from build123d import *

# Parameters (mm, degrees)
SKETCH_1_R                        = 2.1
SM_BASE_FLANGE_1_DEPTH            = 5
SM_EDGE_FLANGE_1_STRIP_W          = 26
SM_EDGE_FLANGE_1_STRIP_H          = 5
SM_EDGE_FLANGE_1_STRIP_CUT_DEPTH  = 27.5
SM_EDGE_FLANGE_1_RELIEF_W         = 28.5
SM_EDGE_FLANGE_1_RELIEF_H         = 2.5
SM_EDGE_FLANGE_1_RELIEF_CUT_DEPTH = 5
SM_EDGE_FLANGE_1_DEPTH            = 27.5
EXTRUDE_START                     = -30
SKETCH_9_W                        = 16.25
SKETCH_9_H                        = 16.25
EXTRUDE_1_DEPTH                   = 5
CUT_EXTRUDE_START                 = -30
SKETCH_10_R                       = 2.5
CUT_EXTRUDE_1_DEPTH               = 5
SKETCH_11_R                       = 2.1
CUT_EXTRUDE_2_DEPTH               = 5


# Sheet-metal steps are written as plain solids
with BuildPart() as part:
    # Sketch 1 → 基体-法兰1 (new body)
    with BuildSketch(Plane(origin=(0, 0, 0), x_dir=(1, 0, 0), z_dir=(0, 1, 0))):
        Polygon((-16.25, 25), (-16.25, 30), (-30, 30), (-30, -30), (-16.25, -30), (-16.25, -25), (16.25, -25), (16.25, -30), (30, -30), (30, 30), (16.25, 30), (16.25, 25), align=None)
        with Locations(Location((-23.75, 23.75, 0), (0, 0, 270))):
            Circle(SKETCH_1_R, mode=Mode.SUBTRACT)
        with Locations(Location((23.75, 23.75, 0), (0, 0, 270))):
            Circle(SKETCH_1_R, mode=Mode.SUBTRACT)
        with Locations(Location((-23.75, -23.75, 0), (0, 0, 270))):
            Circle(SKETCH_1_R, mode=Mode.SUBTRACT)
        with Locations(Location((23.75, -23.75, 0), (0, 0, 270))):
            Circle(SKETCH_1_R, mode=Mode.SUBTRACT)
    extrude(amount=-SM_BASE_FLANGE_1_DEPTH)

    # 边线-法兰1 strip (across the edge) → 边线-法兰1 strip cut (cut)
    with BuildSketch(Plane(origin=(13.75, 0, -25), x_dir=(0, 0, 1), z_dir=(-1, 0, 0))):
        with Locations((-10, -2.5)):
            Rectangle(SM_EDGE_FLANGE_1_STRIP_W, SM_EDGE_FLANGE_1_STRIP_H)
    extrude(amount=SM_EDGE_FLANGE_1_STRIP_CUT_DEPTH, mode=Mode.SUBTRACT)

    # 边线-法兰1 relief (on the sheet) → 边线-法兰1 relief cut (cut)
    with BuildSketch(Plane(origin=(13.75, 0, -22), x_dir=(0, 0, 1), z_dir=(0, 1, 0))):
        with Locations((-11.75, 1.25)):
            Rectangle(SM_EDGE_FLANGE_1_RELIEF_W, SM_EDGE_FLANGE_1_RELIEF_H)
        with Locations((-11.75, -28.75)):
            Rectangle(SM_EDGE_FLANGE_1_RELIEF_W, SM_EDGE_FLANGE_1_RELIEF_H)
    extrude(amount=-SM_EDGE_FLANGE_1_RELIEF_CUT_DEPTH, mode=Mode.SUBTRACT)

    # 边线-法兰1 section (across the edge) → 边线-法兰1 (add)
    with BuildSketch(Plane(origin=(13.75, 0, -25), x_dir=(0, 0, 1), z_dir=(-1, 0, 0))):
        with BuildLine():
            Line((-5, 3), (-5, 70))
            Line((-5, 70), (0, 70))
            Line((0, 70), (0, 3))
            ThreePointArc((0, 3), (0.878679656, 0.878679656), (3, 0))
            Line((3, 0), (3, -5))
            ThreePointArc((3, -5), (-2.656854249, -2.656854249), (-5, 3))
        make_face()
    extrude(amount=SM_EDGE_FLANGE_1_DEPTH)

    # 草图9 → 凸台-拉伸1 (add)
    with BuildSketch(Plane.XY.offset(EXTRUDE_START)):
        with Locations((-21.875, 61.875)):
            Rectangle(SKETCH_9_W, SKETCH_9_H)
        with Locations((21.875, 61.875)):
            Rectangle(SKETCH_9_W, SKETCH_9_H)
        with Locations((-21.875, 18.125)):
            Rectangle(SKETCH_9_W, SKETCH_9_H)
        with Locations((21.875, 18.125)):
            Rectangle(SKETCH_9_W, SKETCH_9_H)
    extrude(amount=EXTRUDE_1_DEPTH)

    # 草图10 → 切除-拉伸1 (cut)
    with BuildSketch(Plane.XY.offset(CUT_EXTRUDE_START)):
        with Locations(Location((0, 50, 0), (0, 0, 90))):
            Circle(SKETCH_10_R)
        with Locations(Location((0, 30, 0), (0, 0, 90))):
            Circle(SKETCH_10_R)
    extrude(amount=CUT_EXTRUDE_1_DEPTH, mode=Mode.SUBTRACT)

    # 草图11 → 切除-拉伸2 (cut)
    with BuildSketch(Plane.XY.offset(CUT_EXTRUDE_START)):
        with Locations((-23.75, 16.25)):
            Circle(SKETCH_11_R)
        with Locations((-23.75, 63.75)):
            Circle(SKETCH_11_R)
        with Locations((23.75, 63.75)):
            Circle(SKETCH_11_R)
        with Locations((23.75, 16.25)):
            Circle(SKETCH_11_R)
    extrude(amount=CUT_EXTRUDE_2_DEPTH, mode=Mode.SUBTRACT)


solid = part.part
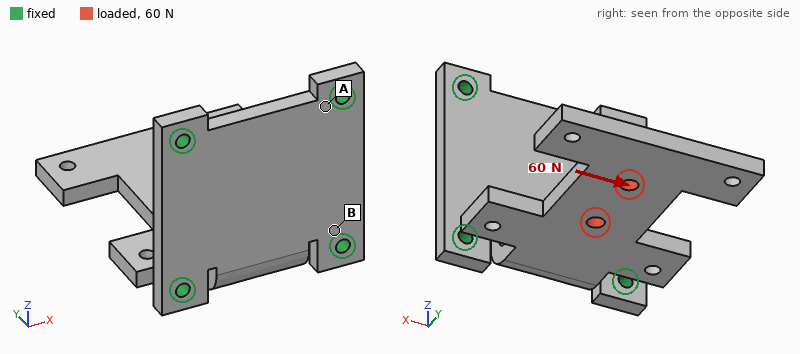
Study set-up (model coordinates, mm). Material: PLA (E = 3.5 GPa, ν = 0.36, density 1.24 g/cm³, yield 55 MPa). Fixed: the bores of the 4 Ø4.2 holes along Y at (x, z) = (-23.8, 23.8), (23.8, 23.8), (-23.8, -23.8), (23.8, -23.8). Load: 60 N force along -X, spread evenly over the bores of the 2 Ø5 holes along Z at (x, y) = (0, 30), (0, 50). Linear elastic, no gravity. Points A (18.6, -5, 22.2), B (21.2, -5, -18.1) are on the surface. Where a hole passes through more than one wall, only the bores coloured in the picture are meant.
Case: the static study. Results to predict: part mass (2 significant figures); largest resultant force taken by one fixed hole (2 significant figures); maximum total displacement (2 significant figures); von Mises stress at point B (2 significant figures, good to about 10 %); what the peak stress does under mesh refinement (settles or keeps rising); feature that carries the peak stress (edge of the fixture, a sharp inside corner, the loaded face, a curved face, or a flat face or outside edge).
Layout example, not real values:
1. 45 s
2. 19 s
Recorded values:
1. 38 g
2. 74 N
3. 1.1 mm
4. 3.7 MPa
5. keeps rising
6. a sharp inside corner
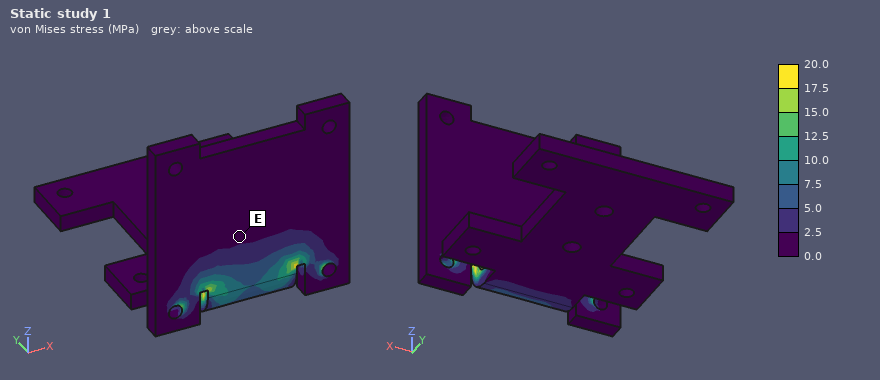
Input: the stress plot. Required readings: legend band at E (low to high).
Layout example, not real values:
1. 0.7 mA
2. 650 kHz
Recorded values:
1. 0.0 to 2.5 MPa
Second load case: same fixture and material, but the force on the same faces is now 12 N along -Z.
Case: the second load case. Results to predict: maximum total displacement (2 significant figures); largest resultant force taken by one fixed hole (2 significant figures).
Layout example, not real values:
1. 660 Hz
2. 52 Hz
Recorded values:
1. 1.1 mm
2. 7.1 N
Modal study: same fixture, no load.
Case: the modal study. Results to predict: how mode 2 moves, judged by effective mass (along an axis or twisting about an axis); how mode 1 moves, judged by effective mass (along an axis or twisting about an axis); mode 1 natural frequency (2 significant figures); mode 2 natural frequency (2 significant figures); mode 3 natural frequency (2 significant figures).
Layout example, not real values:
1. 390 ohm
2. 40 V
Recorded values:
1. along X
2. along Z
3. 150 Hz
4. 330 Hz
5. 550 Hz
